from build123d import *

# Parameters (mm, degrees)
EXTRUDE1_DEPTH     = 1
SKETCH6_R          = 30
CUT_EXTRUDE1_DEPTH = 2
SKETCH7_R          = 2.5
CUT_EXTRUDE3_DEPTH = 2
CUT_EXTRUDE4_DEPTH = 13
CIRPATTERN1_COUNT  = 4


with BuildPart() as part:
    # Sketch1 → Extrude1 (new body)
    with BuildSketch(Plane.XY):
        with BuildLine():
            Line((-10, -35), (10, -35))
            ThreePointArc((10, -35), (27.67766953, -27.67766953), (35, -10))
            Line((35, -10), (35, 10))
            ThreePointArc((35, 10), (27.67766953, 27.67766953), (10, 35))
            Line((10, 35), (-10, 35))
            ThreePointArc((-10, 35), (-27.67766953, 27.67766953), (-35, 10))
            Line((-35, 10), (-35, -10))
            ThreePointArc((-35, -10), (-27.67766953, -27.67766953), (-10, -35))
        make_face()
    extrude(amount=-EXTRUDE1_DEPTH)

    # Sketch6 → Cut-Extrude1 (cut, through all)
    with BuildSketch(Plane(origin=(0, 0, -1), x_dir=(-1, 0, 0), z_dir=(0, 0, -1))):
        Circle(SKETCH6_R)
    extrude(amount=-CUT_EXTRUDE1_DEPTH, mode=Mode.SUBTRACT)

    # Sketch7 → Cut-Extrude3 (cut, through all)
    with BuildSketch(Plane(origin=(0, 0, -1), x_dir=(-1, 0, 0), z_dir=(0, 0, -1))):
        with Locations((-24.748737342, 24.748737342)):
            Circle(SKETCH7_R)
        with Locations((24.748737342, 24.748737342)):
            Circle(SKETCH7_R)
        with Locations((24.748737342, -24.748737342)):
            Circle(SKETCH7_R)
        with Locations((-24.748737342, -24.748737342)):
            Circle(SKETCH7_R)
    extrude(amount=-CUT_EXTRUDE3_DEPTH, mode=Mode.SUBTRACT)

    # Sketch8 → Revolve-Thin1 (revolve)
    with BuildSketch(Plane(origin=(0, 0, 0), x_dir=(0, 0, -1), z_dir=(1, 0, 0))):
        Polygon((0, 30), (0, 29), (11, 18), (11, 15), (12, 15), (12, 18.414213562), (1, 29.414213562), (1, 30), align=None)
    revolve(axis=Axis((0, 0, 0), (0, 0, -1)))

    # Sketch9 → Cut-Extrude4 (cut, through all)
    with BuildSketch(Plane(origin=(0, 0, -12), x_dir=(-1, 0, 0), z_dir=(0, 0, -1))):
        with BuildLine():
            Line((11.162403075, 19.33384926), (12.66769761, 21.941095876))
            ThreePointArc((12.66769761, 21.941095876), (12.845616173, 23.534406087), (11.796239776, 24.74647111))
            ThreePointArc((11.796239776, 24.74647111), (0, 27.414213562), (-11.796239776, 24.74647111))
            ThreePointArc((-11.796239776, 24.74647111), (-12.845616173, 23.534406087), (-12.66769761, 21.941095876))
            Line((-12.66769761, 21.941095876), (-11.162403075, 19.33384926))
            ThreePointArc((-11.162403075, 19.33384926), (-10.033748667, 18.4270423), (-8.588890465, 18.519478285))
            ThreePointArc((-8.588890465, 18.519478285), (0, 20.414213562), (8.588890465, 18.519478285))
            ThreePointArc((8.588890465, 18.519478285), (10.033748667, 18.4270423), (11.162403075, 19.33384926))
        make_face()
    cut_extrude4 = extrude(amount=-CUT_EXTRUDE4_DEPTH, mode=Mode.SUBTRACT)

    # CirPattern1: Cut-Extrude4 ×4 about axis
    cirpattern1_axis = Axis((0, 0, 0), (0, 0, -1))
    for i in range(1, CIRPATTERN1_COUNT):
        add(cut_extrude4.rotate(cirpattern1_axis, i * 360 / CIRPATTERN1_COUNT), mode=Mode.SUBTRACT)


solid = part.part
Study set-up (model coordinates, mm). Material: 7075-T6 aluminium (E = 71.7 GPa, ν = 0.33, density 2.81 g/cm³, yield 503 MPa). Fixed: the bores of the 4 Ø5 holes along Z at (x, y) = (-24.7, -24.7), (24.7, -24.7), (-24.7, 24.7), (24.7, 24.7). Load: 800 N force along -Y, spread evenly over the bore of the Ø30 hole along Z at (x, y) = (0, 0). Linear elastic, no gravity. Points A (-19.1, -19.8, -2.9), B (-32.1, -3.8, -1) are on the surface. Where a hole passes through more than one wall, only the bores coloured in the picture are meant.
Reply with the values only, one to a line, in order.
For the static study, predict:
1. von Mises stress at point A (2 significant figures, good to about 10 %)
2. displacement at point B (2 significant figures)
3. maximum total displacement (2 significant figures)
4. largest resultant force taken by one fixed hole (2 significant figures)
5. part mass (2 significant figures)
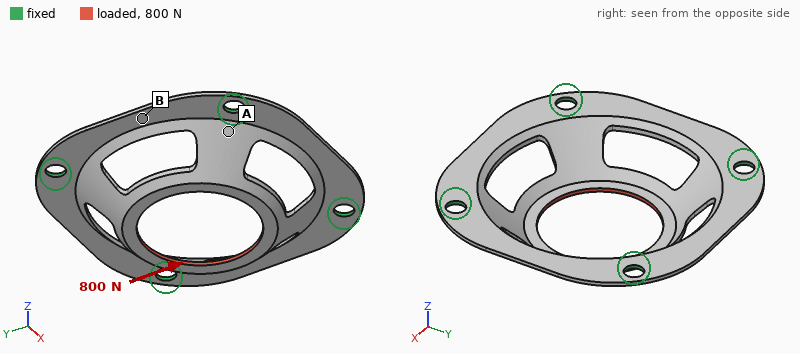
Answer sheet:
82 MPa
0.021 mm
0.14 mm
220 N
9.2 g
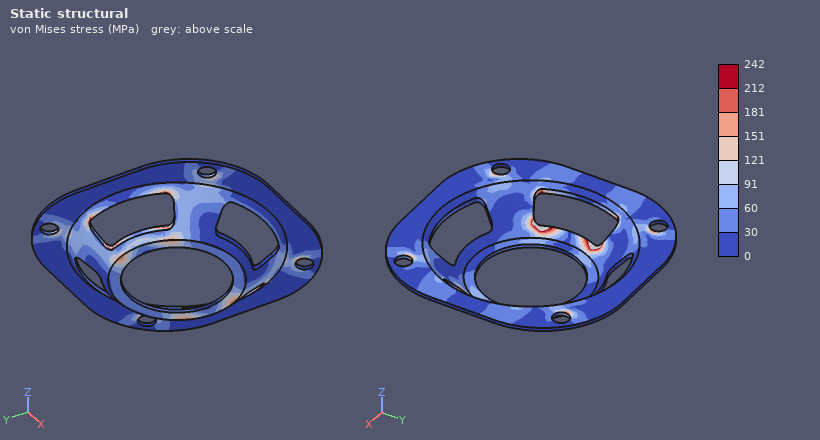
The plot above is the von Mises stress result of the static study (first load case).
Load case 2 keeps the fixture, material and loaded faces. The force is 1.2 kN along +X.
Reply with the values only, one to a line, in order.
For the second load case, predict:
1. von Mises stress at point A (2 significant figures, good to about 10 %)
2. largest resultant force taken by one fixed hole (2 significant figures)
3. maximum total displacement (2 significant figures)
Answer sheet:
120 MPa
330 N
0.21 mm
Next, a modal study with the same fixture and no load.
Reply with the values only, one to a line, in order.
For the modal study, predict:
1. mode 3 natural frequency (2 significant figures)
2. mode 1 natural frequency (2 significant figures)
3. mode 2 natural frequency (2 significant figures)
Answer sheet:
4600 Hz
4500 Hz
4600 Hz
